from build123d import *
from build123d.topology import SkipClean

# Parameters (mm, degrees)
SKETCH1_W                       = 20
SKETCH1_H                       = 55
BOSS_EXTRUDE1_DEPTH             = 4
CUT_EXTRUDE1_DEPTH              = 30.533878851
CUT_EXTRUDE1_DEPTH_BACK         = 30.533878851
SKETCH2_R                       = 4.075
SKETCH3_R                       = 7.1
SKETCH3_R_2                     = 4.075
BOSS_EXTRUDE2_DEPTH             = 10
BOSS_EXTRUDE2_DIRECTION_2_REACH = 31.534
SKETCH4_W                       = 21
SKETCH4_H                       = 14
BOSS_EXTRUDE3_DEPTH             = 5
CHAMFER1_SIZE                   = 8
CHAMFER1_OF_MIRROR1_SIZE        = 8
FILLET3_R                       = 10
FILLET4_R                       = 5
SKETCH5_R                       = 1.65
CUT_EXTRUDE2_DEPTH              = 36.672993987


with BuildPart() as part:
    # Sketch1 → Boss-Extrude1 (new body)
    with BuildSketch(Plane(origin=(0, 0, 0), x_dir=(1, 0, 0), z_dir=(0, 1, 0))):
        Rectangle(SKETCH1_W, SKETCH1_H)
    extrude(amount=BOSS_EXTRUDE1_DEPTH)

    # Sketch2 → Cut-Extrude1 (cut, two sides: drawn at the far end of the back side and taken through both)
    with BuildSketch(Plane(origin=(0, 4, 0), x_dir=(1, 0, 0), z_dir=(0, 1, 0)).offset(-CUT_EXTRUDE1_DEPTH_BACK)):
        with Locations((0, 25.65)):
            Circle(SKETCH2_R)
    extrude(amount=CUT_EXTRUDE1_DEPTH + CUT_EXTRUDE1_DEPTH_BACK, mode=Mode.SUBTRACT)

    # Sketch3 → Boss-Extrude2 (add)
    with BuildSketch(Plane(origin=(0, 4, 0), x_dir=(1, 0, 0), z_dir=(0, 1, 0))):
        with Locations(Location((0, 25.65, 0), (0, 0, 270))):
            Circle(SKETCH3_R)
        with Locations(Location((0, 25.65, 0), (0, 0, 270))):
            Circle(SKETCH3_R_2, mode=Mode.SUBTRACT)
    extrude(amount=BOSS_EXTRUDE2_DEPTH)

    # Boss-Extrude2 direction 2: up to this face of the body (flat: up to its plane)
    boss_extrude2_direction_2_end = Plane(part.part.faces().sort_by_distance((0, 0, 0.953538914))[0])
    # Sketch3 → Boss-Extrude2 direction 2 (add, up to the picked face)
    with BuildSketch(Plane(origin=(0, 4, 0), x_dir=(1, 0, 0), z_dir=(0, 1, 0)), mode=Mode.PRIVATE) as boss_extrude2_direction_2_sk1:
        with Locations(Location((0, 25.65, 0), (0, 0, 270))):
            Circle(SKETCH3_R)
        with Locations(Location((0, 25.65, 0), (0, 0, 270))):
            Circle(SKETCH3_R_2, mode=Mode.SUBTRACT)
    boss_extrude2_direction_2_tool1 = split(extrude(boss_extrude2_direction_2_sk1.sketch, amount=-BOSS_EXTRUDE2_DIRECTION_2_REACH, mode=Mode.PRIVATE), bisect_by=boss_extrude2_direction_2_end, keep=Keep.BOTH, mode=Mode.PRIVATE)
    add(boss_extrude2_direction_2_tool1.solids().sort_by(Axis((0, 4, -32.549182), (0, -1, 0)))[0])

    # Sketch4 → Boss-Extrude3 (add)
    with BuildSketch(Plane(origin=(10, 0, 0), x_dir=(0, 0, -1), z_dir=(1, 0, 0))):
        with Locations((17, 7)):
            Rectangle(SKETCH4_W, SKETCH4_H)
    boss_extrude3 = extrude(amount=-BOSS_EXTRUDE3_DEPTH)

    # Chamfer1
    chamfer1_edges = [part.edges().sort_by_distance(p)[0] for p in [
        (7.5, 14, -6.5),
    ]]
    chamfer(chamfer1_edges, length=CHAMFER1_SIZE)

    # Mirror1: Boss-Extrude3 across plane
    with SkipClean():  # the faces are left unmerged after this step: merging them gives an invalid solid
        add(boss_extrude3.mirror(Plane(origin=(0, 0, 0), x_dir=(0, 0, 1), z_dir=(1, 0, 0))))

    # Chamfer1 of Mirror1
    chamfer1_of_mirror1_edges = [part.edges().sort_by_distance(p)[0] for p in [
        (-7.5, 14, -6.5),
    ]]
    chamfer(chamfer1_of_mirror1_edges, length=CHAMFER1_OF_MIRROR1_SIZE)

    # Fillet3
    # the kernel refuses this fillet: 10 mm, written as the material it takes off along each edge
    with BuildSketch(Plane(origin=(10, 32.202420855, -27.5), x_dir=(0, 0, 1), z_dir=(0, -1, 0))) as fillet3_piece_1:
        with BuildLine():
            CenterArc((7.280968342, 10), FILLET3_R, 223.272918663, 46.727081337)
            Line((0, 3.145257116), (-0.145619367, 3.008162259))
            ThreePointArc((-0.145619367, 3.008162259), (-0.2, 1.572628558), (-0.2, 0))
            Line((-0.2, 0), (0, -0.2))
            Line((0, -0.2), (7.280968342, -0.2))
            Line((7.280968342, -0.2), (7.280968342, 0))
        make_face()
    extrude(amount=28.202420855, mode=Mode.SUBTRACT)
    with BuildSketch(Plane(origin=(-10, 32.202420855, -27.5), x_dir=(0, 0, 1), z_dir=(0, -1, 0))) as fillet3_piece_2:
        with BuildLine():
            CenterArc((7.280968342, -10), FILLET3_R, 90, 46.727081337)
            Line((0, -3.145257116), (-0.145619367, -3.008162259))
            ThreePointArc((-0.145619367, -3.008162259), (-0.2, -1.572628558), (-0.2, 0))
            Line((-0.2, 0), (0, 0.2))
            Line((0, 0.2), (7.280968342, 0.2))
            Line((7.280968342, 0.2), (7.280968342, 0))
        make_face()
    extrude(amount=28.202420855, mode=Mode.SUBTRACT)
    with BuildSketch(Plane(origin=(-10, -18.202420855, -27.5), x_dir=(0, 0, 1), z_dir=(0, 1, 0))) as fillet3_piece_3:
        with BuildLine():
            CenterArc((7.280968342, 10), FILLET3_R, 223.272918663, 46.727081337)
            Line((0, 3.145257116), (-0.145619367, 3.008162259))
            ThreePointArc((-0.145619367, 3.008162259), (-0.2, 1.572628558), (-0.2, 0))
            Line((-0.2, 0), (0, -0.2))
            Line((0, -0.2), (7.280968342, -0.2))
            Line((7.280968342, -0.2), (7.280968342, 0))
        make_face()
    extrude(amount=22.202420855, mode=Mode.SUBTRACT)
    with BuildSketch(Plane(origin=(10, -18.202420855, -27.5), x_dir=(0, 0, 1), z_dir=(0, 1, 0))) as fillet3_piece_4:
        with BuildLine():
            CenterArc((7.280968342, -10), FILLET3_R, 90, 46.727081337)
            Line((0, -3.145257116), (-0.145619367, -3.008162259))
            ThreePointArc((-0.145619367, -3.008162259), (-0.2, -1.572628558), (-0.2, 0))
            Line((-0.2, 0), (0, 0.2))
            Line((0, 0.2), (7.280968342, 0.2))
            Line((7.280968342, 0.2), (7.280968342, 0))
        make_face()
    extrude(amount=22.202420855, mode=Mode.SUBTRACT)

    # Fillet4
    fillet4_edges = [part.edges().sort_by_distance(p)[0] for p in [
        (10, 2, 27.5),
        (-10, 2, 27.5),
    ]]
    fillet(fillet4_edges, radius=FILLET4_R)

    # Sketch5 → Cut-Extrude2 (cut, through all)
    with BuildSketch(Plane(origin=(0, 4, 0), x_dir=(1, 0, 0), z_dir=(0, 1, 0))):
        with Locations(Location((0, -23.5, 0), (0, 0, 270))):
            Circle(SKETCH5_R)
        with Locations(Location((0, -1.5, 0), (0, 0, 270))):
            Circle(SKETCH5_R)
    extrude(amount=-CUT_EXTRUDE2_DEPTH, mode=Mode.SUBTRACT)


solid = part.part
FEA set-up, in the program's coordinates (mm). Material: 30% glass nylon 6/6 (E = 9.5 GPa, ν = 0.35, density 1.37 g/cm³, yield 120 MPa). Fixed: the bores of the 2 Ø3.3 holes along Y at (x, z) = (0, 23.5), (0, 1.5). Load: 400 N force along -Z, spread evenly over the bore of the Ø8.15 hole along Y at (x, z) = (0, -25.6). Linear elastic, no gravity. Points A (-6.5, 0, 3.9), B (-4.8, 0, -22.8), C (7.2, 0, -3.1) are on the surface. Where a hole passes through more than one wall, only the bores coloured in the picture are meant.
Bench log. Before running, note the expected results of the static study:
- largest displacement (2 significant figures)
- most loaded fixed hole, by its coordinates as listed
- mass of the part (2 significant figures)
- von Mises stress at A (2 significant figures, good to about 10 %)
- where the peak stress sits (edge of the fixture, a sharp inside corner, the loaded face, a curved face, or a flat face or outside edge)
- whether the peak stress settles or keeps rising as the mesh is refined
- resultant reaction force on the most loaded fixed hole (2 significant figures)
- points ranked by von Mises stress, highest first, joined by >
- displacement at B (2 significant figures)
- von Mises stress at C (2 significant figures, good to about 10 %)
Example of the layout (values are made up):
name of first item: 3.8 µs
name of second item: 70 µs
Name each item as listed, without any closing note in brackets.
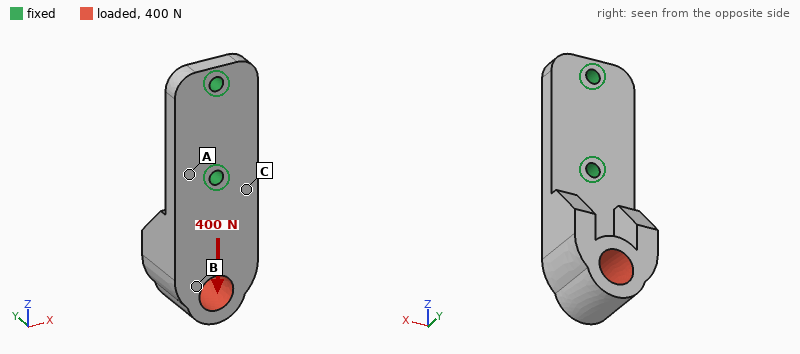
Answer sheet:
largest displacement: 0.70 mm
most loaded fixed hole, by its coordinates as listed: (0, 1.5)
mass of the part: 9.2 g
von Mises stress at A: 9.3 MPa
where the peak stress sits: edge of the fixture
whether the peak stress settles or keeps rising as the mesh is refined: keeps rising
resultant reaction force on the most loaded fixed hole: 330 N
points ranked by von Mises stress, highest first, joined by >: C > A > B
displacement at B: 0.42 mm
von Mises stress at C: 29 MPa
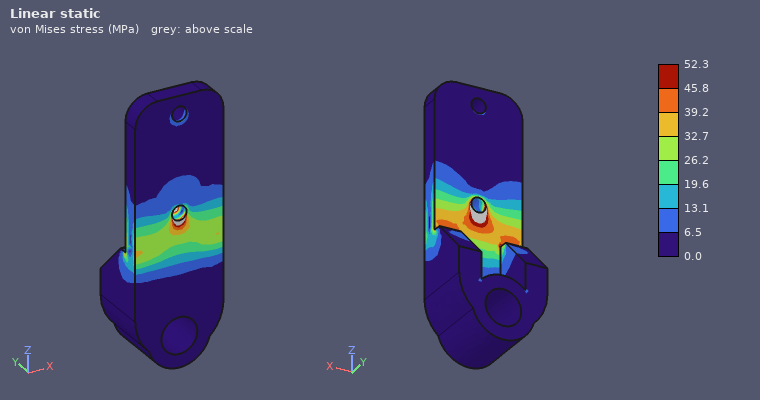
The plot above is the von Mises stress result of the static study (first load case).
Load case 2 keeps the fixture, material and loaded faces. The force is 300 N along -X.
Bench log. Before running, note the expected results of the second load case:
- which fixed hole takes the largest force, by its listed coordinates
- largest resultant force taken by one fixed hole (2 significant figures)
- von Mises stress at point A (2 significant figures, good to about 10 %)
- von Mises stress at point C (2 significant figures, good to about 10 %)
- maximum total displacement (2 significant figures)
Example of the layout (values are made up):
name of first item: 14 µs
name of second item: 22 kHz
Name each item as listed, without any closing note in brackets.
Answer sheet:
which fixed hole takes the largest force, by its listed coordinates: (0, 1.5)
largest resultant force taken by one fixed hole: 590 N
von Mises stress at point A: 25 MPa
von Mises stress at point C: 17 MPa
maximum total displacement: 0.35 mm
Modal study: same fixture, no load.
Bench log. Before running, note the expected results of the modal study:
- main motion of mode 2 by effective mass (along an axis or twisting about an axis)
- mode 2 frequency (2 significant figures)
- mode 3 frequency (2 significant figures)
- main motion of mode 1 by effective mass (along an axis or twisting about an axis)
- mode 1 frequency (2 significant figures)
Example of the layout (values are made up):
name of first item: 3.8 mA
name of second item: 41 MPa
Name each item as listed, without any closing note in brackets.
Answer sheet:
main motion of mode 2 by effective mass: along X
mode 2 frequency: 2600 Hz
mode 3 frequency: 4100 Hz
main motion of mode 1 by effective mass: along Y
mode 1 frequency: 1100 Hz
